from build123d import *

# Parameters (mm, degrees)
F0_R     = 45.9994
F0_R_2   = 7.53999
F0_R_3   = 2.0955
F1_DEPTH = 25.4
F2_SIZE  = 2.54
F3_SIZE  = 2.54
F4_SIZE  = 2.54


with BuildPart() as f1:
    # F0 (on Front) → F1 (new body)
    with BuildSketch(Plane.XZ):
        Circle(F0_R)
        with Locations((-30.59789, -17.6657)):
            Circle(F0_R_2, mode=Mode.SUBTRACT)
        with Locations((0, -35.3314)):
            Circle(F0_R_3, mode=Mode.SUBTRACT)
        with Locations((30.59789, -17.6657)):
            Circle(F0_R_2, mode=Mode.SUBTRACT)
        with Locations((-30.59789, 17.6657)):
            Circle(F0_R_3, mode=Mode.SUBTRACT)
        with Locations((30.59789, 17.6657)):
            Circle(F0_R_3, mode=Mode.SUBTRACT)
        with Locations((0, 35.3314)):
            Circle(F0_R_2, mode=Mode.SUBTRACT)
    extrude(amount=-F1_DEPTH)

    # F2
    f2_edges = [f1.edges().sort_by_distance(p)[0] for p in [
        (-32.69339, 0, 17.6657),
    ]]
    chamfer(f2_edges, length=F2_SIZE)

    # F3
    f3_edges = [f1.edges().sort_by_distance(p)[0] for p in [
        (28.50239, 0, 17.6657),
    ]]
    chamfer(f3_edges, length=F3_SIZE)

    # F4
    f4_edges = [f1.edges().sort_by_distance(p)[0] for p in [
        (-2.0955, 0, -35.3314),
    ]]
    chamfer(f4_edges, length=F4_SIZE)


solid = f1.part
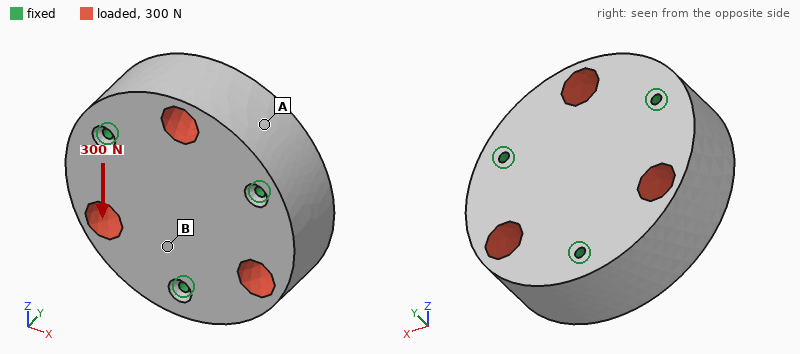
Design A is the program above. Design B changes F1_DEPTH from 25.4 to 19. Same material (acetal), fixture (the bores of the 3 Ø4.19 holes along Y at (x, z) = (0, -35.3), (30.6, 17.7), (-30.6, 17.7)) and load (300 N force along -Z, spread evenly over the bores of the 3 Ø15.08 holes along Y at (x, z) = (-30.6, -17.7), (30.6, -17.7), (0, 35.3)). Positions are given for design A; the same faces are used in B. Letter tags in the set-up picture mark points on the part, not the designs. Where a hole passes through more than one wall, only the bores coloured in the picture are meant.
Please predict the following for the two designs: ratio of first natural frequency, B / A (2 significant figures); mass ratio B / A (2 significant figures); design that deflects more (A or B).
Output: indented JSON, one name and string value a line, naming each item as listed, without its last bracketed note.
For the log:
{
  "ratio of first natural frequency, B / A": "0.84",
  "mass ratio B / A": "0.75",
  "design that deflects more": "B"
}
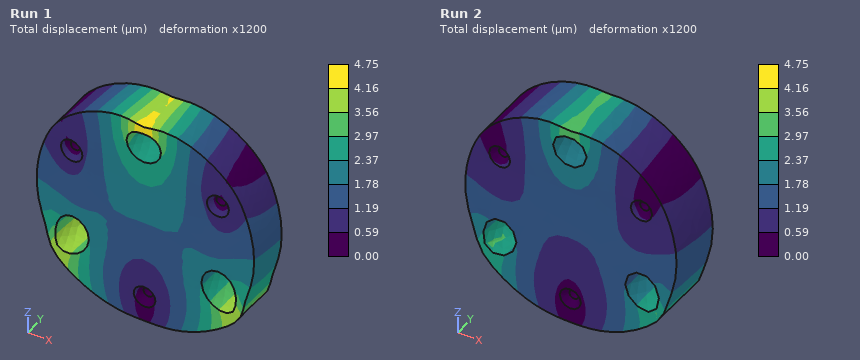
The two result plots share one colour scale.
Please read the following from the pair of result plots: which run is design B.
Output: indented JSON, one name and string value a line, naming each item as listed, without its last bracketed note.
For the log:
{
  "which run is design B": "Run 1"
}
